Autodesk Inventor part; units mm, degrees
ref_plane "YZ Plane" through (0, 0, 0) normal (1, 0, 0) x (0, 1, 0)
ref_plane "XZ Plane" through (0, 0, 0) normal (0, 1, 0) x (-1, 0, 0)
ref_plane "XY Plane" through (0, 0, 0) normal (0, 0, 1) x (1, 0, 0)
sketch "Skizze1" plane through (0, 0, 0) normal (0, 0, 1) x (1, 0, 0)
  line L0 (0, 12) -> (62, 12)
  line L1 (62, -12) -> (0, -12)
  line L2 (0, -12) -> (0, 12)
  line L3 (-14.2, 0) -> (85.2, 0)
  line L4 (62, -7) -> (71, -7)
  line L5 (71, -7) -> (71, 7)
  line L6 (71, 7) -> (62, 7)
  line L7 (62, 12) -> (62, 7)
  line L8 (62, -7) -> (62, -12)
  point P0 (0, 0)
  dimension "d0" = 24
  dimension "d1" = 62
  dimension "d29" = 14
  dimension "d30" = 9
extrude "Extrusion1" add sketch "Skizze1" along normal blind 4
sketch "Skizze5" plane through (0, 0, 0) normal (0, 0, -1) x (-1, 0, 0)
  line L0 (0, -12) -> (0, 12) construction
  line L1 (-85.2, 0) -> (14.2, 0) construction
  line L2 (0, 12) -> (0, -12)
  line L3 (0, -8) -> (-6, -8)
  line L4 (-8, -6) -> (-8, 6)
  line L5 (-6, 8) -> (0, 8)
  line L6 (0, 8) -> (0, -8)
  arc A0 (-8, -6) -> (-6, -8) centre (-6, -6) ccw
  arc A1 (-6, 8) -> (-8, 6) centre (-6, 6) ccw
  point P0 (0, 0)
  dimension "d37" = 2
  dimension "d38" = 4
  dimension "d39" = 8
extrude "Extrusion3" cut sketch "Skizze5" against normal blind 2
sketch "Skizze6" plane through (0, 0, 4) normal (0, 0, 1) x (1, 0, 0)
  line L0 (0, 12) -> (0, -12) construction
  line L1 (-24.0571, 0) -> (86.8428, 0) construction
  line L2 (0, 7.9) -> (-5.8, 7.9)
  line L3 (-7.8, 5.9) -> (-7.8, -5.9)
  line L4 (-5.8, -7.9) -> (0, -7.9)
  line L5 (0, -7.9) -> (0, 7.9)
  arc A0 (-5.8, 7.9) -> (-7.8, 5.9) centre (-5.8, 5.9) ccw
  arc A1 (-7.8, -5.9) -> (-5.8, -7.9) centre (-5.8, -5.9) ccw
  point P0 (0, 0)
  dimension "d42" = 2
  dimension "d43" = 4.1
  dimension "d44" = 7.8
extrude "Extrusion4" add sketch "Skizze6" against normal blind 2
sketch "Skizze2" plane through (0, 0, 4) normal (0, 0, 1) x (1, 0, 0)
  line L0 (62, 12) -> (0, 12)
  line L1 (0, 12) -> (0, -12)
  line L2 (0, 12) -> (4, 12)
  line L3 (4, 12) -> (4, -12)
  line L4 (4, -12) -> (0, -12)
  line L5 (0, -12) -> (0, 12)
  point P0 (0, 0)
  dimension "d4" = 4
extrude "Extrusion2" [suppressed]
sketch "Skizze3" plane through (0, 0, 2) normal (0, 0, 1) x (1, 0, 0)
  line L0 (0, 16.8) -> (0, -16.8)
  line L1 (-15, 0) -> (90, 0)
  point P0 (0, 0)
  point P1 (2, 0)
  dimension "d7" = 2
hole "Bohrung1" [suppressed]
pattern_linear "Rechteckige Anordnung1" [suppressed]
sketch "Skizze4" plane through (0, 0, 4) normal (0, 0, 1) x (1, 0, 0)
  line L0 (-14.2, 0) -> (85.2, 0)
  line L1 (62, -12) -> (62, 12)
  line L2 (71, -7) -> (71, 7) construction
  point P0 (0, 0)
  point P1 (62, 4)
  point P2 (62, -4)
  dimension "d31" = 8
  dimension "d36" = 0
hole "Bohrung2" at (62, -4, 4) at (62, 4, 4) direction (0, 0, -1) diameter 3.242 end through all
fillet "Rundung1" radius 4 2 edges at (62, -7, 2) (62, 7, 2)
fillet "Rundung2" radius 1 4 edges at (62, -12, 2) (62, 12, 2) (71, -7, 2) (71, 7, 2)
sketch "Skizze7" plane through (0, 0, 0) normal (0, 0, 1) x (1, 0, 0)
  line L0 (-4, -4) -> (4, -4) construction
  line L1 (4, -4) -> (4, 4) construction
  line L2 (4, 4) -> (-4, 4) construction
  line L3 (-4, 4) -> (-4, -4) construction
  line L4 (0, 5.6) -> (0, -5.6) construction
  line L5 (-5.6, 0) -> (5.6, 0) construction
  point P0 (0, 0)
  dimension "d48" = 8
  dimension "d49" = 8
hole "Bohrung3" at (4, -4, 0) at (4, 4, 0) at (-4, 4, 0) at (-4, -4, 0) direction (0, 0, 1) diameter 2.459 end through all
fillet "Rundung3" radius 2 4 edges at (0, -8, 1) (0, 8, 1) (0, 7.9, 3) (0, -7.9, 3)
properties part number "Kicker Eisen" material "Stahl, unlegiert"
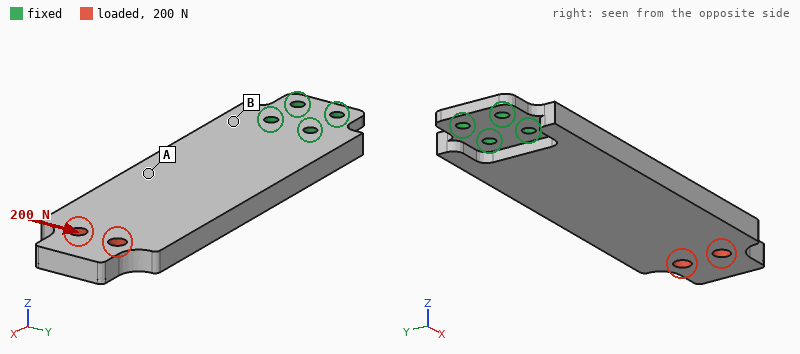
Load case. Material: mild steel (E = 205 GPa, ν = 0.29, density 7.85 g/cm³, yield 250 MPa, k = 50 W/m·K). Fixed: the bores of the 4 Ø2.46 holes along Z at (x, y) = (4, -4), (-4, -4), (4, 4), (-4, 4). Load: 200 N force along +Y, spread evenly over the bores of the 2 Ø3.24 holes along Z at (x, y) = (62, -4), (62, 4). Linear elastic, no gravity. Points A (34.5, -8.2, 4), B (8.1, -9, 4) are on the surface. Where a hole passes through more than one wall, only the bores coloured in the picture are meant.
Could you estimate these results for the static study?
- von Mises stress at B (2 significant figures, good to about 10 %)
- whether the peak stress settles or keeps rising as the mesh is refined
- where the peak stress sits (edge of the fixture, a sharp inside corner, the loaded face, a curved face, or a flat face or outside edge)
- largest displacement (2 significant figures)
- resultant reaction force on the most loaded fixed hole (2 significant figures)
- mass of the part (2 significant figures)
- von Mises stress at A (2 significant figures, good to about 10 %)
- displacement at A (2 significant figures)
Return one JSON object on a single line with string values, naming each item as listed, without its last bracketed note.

{"von Mises stress at B": "27 MPa", "whether the peak stress settles or keeps rising as the mesh is refined": "keeps rising", "where the peak stress sits": "edge of the fixture", "largest displacement": "36 µm", "resultant reaction force on the most loaded fixed hole": "730 N", "mass of the part": "50 g", "von Mises stress at A": "10 MPa", "displacement at A": "15 µm"}
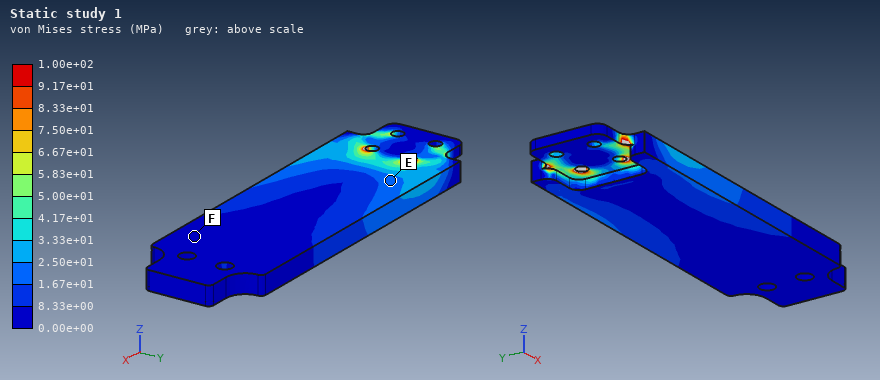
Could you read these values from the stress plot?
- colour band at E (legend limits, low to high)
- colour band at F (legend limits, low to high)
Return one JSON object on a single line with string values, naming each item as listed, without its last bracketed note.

{"colour band at E": "1.67e+01 to 2.50e+01 MPa", "colour band at F": "0.00e+00 to 8.33e+00 MPa"}
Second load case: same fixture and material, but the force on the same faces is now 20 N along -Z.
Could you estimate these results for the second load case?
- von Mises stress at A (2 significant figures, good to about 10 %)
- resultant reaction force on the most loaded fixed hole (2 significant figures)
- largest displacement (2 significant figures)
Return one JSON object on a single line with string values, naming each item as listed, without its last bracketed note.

{"von Mises stress at A": "8.6 MPa", "resultant reaction force on the most loaded fixed hole": "50 N", "largest displacement": "0.10 mm"}
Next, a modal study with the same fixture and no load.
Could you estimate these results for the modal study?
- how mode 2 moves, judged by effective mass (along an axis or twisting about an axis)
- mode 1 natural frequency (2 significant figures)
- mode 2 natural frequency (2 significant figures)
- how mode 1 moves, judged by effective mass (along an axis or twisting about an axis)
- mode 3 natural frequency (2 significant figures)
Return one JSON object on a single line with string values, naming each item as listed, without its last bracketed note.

{"how mode 2 moves, judged by effective mass": "along Y", "mode 1 natural frequency": "600 Hz", "mode 2 natural frequency": "3100 Hz", "how mode 1 moves, judged by effective mass": "along Z", "mode 3 natural frequency": "3800 Hz"}
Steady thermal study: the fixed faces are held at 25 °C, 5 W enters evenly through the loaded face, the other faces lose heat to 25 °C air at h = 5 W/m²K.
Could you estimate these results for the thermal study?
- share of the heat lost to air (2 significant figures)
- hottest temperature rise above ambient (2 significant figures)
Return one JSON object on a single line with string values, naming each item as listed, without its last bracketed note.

{"share of the heat lost to air": "13 %", "hottest temperature rise above ambient": "64 K"}
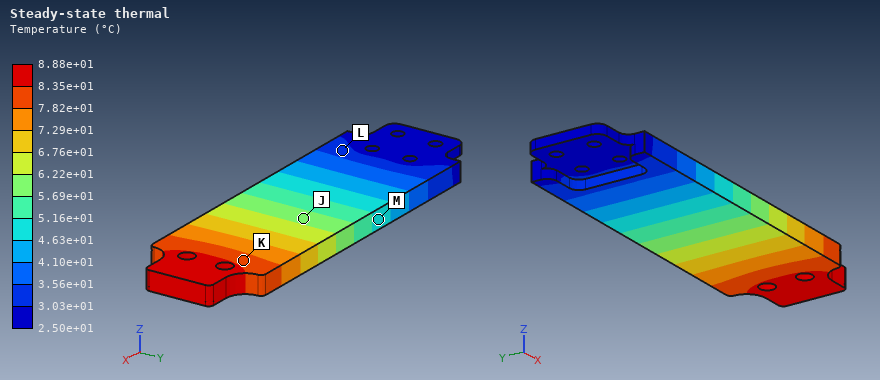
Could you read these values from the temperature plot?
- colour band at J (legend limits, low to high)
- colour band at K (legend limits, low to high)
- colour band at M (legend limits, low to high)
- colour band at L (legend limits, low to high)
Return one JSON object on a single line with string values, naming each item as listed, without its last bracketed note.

{"colour band at J": "5.69e+01 to 6.22e+01 °C", "colour band at K": "7.82e+01 to 8.35e+01 °C", "colour band at M": "4.63e+01 to 5.16e+01 °C", "colour band at L": "3.03e+01 to 3.56e+01 °C"}
